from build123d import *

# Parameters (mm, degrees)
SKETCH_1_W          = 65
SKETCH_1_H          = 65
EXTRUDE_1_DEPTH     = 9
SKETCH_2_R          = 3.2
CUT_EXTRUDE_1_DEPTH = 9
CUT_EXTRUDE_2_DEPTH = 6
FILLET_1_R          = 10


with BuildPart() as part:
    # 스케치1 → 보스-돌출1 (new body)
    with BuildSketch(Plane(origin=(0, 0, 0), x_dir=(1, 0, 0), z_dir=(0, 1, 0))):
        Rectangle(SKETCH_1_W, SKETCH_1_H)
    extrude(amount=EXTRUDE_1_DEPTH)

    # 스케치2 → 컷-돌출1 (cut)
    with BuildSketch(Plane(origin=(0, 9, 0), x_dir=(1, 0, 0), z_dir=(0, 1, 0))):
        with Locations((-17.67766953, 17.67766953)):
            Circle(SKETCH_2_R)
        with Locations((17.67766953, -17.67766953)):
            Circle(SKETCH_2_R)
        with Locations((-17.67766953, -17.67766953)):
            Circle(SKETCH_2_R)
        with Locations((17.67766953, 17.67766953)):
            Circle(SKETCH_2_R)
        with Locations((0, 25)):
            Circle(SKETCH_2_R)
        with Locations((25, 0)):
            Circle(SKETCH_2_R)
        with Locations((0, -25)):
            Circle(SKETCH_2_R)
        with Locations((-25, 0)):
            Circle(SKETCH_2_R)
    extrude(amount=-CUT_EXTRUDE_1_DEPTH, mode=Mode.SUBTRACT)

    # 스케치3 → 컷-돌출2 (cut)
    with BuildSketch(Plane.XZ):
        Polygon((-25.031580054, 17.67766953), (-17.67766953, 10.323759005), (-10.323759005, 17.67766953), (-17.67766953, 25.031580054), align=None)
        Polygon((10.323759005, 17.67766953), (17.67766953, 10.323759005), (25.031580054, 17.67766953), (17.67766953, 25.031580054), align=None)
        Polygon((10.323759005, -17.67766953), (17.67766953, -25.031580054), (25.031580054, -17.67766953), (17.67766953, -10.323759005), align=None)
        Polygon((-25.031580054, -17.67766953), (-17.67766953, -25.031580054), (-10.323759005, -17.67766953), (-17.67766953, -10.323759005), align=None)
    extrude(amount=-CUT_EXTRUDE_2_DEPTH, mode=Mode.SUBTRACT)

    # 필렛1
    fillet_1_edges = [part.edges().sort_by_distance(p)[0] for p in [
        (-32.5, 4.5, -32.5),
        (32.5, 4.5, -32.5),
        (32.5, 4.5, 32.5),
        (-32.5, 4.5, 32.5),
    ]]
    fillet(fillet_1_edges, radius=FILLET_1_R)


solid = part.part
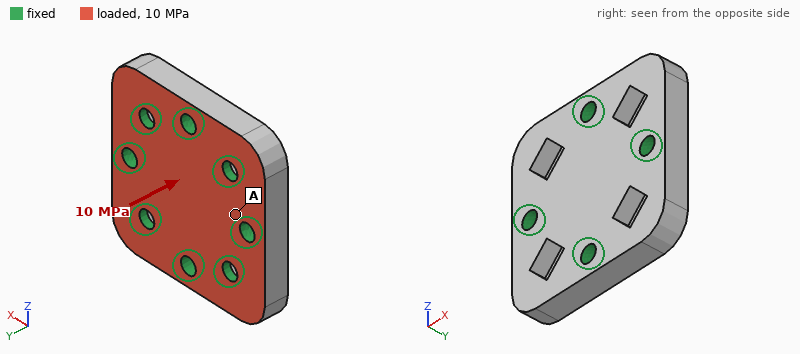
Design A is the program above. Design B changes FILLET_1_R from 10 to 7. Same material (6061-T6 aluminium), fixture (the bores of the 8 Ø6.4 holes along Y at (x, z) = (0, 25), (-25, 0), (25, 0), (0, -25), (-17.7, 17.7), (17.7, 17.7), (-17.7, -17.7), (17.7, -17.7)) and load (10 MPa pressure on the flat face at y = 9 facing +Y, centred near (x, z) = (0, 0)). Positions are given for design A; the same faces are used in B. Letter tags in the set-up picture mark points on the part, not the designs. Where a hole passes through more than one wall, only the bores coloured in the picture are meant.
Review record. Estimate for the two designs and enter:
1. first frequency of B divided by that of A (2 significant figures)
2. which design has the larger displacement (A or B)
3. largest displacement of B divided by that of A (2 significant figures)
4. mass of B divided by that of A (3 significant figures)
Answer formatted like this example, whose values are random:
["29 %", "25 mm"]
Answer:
["0.94", "B", "1.2", "1.01"]
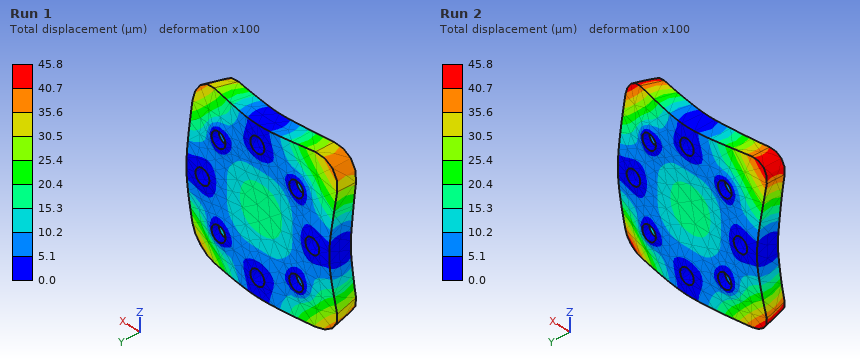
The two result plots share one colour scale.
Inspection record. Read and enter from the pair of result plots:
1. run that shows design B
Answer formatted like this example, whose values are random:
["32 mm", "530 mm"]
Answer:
["Run 2"]
